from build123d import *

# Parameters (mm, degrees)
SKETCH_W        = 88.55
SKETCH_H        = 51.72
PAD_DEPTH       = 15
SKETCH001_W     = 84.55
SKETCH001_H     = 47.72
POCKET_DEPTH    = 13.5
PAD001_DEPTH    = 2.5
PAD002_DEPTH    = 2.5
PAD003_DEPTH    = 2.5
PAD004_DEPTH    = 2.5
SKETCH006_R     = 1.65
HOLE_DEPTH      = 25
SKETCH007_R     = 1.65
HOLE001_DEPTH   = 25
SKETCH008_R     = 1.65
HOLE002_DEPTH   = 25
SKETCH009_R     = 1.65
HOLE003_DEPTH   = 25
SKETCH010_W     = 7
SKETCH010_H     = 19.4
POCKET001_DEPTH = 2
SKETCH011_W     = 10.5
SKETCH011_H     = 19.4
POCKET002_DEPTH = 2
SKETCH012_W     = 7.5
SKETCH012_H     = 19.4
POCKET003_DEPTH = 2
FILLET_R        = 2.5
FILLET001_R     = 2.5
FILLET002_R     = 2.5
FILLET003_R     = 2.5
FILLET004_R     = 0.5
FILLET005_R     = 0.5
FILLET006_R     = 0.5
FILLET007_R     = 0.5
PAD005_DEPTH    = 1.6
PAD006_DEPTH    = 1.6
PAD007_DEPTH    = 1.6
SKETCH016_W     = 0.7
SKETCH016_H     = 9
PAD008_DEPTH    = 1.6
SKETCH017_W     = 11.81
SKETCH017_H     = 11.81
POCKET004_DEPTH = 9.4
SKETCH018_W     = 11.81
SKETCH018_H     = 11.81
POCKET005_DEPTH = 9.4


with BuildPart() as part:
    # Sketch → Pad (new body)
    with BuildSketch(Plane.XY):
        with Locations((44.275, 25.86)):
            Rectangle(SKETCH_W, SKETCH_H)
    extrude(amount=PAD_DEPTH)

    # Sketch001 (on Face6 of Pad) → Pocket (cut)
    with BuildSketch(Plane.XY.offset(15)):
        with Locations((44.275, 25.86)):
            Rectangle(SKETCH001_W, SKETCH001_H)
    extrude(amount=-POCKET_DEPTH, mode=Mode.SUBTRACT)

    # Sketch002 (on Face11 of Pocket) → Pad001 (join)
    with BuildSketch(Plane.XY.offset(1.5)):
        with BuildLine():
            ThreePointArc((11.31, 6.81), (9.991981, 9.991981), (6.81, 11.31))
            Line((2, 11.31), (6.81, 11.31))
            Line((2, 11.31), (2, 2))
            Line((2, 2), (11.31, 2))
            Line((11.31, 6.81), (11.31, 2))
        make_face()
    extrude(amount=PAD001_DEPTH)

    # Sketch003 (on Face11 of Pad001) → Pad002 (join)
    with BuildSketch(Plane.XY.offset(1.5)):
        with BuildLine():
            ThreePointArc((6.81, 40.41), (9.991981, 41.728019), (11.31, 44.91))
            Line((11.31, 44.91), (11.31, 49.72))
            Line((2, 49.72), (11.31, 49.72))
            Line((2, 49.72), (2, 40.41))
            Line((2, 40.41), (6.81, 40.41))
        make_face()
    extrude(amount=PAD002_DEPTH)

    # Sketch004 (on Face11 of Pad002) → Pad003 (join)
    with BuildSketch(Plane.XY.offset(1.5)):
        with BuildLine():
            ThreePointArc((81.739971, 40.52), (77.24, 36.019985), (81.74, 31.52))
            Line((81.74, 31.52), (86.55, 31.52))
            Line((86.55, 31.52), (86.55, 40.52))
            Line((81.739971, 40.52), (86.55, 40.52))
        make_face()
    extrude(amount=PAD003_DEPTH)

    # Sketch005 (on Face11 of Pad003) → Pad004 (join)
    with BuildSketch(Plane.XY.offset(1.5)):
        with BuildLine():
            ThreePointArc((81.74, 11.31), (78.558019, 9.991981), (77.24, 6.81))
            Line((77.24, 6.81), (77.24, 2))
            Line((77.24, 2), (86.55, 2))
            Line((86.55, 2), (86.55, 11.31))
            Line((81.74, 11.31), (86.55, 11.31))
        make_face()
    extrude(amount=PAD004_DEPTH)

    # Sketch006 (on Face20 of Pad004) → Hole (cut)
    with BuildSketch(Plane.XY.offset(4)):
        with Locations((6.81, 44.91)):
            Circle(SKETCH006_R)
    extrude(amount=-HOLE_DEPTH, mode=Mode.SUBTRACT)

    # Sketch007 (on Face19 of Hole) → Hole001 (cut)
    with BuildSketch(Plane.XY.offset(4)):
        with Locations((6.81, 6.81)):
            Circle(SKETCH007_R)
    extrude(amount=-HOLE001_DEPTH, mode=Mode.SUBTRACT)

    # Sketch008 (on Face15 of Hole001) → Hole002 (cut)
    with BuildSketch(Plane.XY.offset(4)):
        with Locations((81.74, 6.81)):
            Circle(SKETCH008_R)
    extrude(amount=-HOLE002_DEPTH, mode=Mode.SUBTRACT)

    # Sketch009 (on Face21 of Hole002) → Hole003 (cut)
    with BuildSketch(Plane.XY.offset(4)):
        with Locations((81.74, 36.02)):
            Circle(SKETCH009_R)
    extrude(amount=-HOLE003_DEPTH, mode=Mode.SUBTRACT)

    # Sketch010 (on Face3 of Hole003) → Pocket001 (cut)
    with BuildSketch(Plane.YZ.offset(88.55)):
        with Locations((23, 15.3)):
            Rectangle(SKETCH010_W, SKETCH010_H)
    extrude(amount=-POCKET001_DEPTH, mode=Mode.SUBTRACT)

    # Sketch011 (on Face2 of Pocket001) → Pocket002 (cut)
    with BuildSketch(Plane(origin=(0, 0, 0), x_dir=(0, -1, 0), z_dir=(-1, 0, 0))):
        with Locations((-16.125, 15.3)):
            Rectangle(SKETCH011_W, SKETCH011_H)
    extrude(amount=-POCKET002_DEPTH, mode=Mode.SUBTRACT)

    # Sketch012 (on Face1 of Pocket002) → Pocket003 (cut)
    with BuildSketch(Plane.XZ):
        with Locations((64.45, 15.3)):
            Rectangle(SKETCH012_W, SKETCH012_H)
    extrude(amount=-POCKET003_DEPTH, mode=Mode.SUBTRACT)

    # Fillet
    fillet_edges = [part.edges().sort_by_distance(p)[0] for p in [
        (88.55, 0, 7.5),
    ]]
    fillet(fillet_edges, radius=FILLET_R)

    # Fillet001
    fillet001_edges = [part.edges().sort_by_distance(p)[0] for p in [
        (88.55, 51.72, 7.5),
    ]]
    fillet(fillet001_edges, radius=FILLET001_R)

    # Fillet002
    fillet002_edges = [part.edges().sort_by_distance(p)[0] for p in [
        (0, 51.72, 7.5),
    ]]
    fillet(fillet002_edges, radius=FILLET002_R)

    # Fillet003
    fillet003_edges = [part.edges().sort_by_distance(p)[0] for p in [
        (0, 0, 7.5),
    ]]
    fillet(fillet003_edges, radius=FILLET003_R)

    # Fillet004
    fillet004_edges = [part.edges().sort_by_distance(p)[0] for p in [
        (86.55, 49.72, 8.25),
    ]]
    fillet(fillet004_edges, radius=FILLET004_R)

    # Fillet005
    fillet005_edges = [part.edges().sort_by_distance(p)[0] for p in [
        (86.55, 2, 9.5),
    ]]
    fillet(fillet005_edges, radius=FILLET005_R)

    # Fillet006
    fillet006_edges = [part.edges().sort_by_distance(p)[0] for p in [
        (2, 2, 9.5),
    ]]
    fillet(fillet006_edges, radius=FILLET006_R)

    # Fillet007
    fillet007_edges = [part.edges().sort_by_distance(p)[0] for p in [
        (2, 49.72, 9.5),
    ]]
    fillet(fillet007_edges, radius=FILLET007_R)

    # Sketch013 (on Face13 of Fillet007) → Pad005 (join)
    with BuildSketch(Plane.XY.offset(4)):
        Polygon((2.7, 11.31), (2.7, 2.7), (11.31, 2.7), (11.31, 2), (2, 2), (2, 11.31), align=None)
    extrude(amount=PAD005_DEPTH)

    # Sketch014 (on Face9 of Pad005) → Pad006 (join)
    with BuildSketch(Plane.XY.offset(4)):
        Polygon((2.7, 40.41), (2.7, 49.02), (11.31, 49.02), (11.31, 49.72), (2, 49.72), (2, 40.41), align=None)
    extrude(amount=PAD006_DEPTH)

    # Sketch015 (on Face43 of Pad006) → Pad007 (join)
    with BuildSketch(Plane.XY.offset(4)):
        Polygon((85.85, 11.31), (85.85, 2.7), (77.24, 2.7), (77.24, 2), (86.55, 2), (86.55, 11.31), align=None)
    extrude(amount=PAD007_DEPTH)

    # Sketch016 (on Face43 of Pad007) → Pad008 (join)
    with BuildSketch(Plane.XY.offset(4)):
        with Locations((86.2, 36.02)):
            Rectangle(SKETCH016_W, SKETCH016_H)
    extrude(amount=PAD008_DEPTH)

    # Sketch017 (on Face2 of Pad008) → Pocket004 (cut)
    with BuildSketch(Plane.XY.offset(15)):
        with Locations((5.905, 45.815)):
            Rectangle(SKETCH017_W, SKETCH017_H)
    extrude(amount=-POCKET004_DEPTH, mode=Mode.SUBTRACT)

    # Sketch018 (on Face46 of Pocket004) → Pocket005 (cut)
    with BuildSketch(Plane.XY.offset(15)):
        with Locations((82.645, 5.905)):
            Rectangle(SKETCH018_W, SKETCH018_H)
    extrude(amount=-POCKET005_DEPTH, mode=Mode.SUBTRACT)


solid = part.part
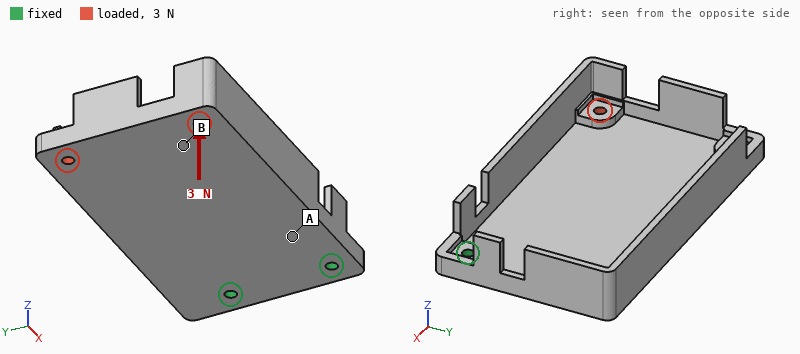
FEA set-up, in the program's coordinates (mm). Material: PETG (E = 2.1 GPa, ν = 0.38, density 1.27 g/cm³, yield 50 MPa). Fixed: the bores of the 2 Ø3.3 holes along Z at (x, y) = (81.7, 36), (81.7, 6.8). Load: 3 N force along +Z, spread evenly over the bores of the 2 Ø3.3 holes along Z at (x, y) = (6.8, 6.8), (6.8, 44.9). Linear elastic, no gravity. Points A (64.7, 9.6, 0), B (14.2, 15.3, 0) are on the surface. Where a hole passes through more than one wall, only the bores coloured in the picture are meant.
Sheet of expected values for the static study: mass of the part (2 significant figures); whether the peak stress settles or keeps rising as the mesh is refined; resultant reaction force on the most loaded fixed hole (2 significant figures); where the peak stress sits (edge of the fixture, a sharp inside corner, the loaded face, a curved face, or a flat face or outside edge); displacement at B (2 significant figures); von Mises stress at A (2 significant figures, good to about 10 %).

17 g
keeps rising
2.8 N
a sharp inside corner
0.92 mm
1.3 MPa
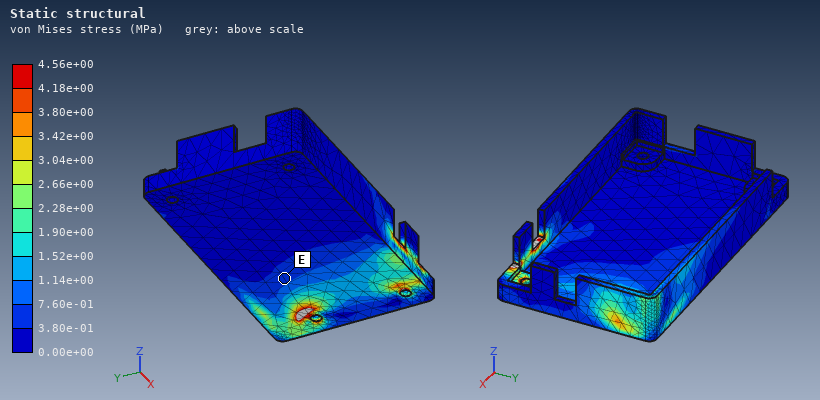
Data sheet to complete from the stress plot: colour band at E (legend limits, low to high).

3.80e-01 to 7.60e-01 MPa
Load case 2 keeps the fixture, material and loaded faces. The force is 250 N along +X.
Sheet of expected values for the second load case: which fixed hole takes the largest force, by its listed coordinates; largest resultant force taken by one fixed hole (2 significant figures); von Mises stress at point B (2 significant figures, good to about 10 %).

(81.7, 36)
160 N
2.3 MPa
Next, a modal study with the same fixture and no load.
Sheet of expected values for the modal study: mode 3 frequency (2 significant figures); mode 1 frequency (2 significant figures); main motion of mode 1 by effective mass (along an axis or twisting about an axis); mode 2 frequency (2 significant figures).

670 Hz
100 Hz
along Z
180 Hz
